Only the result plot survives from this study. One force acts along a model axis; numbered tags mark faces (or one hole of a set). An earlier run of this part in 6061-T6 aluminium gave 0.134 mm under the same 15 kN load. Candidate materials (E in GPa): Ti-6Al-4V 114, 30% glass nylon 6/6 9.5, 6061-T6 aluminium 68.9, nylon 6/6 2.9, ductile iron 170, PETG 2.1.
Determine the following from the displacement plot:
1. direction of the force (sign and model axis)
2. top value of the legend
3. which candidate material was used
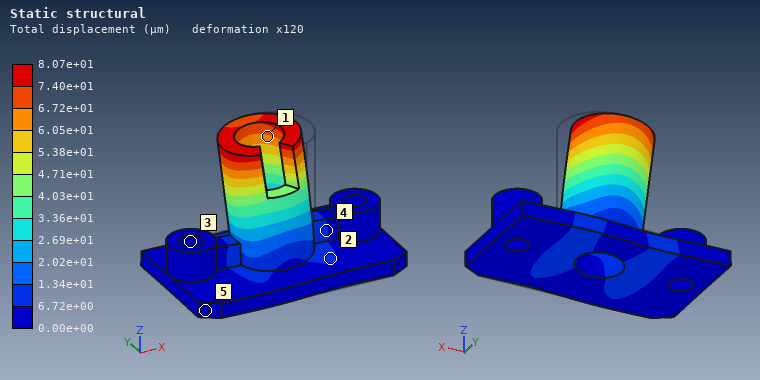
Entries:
-X
8.07e+01 µm
Ti-6Al-4V
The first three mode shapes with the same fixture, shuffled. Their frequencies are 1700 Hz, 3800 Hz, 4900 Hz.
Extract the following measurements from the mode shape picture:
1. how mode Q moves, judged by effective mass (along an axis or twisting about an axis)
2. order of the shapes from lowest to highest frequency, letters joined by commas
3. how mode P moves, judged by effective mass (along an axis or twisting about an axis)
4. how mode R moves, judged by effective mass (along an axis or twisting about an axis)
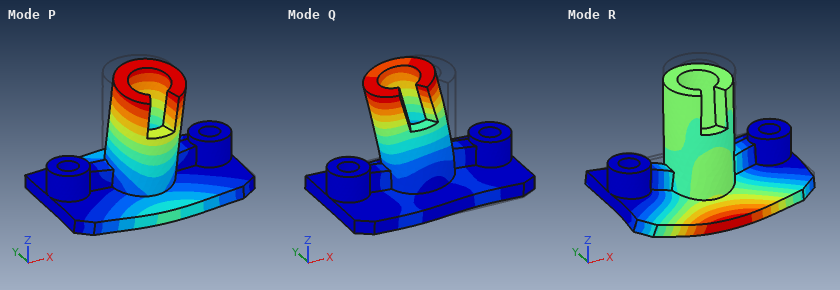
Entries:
along X
P, Q, R
along Y
along Z
